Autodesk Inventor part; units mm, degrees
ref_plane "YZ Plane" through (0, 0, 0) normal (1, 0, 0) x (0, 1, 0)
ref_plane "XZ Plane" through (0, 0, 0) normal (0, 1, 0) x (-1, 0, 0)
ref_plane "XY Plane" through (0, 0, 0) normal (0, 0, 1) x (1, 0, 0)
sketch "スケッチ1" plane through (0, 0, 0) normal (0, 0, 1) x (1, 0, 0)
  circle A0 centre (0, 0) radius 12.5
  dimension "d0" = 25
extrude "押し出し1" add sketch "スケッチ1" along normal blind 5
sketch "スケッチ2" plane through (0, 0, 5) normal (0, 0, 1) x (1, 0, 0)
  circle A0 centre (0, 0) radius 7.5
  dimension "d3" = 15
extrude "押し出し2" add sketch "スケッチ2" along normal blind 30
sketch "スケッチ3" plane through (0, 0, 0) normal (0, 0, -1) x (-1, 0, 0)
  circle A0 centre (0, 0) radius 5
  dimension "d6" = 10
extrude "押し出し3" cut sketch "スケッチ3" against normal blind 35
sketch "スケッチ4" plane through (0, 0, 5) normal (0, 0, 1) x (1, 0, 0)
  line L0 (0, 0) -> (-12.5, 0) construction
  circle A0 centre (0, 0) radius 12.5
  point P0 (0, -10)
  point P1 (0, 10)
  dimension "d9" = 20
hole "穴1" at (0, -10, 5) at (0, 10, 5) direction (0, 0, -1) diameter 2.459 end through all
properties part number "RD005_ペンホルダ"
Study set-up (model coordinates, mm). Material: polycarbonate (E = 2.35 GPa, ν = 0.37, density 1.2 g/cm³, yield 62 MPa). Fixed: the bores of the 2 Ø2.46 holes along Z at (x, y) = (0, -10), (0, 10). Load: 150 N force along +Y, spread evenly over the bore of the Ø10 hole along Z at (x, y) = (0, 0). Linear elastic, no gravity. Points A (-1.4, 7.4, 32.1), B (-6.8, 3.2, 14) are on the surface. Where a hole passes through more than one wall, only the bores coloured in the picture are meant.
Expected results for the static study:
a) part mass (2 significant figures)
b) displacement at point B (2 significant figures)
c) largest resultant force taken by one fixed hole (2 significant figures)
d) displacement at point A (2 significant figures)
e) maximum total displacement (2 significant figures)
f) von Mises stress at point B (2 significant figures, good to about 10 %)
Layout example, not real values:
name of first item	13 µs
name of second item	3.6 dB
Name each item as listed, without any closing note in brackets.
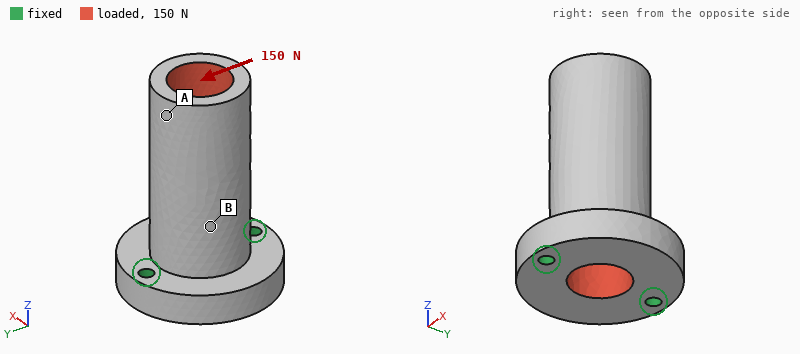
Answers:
part mass	6.0 g
displacement at point B	0.062 mm
largest resultant force taken by one fixed hole	150 N
displacement at point A	0.19 mm
maximum total displacement	0.21 mm
von Mises stress at point B	2.9 MPa
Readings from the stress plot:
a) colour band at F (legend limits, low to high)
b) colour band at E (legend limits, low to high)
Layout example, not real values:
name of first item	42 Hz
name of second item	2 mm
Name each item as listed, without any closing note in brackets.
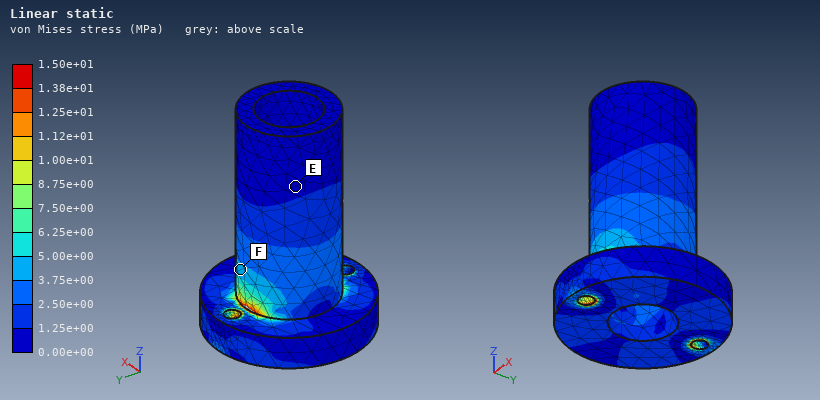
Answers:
colour band at F	3.75e+00 to 5.00e+00 MPa
colour band at E	0.00e+00 to 1.25e+00 MPa
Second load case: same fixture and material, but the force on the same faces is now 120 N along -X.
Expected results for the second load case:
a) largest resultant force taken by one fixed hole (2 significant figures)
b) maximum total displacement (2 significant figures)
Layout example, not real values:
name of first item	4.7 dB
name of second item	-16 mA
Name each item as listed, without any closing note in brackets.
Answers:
largest resultant force taken by one fixed hole	60 N
maximum total displacement	0.54 mm
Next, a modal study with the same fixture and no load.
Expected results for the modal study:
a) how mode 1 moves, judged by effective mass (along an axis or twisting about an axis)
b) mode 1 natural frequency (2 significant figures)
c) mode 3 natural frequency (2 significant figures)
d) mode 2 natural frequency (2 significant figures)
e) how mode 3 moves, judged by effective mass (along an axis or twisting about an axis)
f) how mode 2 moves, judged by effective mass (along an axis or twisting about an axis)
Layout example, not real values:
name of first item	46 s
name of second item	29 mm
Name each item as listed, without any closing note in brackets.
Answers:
how mode 1 moves, judged by effective mass	along X
mode 1 natural frequency	1400 Hz
mode 3 natural frequency	6000 Hz
mode 2 natural frequency	2500 Hz
how mode 3 moves, judged by effective mass	along Z
how mode 2 moves, judged by effective mass	along Y
